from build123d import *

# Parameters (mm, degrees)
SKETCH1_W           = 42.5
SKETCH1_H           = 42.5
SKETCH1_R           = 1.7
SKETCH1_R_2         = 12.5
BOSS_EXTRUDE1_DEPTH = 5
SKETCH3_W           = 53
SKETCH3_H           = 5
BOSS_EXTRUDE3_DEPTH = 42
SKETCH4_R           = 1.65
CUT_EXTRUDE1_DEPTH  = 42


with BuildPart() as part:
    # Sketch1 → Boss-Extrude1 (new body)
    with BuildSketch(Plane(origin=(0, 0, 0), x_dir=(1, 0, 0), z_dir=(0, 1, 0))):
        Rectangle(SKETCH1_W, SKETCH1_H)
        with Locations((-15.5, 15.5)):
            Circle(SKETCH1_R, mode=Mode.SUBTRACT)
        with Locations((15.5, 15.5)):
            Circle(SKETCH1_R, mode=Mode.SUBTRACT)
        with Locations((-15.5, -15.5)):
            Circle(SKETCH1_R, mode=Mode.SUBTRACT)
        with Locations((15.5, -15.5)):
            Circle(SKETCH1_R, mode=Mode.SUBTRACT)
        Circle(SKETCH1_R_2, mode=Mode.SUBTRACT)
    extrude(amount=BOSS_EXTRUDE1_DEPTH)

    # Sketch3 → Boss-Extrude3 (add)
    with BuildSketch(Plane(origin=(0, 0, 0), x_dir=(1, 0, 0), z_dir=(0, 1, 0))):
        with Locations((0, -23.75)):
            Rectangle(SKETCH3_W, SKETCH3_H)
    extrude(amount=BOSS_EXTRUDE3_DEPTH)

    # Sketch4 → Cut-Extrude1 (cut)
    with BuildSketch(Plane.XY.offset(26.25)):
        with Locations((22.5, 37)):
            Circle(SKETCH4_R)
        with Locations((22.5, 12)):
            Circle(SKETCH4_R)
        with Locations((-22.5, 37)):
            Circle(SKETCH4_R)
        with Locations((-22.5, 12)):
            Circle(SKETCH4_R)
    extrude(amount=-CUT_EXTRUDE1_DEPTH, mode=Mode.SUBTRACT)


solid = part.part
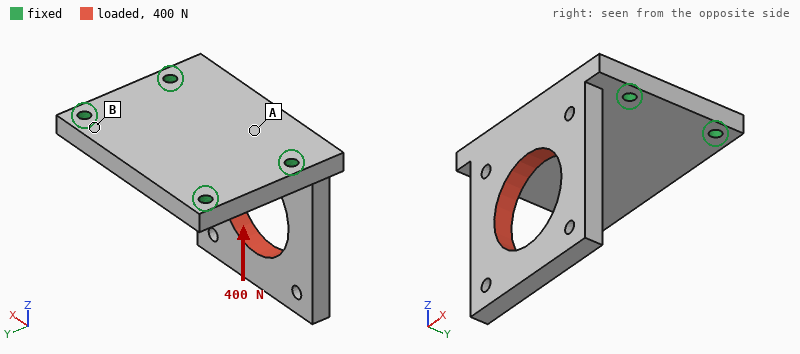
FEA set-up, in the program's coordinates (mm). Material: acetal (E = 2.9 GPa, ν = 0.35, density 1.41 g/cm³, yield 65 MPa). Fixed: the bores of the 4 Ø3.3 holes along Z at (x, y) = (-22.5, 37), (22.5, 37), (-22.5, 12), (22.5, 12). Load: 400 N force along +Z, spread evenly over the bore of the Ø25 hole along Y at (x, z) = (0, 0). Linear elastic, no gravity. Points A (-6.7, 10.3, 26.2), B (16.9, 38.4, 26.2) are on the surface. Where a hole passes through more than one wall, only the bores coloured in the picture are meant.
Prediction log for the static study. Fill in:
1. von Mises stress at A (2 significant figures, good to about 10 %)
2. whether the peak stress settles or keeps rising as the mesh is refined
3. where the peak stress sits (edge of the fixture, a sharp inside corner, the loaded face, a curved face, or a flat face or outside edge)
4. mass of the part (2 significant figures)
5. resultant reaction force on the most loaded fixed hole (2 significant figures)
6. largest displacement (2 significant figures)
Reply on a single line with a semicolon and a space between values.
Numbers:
5.5 MPa; keeps rising; edge of the fixture; 24 g; 230 N; 0.80 mm
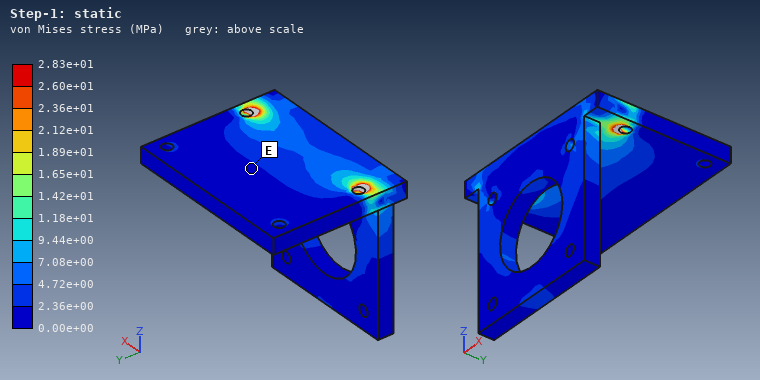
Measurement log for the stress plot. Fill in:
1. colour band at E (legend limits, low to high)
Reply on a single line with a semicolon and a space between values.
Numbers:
0.00e+00 to 2.36e+00 MPa
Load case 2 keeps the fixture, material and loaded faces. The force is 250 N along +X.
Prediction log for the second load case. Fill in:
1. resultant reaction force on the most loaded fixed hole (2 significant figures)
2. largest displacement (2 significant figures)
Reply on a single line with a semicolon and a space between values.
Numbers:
190 N; 0.41 mm
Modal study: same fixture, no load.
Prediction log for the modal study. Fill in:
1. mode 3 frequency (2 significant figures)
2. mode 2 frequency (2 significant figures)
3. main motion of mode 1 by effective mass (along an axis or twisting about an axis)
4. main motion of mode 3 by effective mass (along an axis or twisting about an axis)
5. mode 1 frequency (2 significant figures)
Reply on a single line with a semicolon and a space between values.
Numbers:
1600 Hz; 1100 Hz; along Y; along X; 430 Hz
